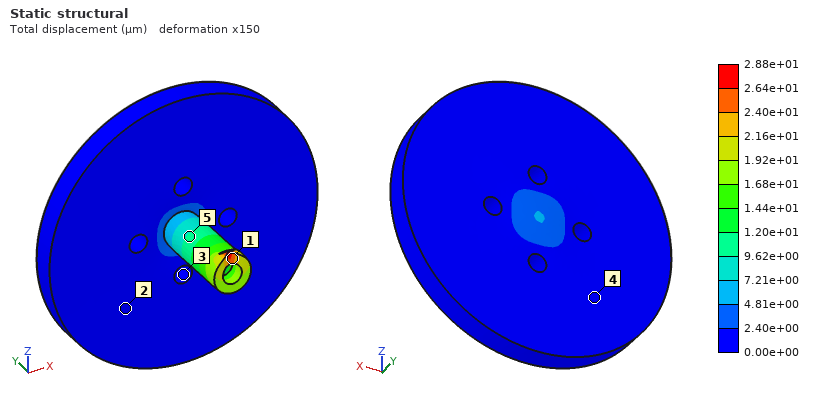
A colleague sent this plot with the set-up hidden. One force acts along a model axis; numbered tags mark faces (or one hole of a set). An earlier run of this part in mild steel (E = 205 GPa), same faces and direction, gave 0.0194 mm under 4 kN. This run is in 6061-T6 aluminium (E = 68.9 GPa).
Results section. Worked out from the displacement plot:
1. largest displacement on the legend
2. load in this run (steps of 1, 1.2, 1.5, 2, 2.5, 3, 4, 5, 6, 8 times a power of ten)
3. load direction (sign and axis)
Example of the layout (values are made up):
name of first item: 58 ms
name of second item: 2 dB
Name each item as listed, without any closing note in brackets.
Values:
largest displacement on the legend: 2.88e+01 µm
load in this run: 2 kN
load direction: +Y
